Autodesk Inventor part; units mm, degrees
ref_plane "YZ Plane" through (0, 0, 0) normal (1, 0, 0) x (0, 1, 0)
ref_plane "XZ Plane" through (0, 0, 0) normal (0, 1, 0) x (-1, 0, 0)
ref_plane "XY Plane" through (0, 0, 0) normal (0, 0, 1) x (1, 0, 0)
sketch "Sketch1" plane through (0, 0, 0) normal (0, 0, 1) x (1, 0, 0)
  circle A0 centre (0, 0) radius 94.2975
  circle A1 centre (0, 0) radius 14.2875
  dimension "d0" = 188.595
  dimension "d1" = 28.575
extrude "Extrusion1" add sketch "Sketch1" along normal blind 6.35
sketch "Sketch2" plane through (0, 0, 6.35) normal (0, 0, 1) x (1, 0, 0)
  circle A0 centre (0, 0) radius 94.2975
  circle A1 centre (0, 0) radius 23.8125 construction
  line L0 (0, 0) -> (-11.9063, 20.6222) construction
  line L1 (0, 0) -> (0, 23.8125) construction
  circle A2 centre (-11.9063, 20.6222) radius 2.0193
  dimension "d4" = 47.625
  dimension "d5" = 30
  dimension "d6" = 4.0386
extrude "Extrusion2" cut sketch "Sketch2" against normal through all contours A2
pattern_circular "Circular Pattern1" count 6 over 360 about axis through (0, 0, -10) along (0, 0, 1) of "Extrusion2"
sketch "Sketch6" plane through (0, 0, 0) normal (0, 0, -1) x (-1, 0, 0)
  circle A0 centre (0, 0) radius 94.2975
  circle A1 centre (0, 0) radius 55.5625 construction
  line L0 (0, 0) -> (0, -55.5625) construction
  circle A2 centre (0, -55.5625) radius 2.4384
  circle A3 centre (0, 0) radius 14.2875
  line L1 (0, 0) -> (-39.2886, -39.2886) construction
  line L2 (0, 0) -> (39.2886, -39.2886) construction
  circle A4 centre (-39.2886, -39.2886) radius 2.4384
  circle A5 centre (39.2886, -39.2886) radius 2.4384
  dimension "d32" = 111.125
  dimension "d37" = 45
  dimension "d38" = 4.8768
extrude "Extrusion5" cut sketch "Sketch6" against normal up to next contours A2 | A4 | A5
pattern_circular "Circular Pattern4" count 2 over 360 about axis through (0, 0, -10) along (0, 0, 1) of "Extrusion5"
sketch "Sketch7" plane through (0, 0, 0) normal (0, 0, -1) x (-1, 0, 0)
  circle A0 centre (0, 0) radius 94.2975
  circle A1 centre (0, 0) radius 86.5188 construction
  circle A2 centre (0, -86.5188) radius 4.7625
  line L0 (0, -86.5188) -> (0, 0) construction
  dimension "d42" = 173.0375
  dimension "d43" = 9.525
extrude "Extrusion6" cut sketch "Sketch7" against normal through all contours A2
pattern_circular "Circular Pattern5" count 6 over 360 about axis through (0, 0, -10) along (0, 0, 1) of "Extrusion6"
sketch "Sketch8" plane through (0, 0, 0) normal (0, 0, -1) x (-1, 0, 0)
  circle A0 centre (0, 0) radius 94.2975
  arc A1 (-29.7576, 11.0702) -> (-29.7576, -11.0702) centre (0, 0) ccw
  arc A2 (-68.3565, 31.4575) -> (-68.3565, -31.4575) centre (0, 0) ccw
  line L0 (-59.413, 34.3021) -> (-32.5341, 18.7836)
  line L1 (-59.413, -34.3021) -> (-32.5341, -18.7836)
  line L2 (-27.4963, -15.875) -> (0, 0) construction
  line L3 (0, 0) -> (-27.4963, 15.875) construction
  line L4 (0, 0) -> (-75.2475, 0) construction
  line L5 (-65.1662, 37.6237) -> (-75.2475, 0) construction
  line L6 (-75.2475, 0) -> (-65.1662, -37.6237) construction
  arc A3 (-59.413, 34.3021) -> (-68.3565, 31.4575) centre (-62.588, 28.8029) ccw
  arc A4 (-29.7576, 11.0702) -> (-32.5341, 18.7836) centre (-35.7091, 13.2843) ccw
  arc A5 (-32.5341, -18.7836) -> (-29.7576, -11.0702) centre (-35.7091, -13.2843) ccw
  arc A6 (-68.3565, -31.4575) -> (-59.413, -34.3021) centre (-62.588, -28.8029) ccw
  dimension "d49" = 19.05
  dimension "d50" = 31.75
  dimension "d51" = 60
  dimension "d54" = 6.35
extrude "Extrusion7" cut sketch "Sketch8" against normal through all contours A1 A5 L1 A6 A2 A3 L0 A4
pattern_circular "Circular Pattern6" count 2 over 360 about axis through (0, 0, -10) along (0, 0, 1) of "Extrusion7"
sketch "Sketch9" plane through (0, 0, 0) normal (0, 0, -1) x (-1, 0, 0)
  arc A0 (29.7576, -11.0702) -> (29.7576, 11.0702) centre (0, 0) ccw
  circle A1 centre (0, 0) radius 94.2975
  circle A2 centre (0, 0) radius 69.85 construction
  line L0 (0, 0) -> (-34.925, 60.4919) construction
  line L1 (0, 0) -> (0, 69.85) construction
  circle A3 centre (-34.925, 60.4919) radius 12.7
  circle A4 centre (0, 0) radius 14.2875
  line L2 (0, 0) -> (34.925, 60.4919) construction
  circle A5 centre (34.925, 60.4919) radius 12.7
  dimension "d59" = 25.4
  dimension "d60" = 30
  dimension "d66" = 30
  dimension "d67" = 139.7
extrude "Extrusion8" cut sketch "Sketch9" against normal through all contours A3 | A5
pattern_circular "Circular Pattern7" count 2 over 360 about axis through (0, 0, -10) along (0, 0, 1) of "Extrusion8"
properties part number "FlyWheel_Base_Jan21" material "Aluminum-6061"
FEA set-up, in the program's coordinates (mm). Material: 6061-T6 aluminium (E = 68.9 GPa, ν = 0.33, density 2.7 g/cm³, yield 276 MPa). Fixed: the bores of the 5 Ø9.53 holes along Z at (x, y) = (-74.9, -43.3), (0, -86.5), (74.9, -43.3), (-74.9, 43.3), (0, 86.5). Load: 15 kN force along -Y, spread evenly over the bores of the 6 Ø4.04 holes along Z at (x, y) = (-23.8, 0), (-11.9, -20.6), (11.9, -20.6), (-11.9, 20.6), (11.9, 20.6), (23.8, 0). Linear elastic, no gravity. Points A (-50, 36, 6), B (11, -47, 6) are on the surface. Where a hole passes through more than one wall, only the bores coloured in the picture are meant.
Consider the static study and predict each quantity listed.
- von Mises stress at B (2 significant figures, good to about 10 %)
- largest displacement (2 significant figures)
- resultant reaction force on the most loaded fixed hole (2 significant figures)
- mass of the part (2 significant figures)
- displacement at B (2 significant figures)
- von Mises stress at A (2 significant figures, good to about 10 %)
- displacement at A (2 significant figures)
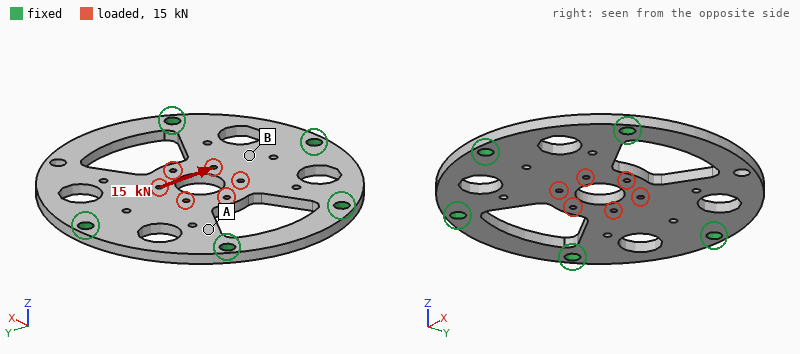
23 MPa
27 µm
5.8 kN
340 g
16 µm
7.1 MPa
8.6 µm
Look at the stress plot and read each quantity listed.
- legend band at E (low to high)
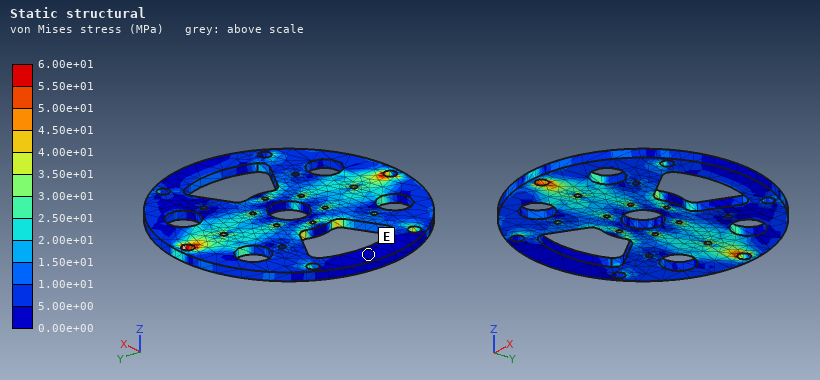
0.00e+00 to 5.00e+00 MPa
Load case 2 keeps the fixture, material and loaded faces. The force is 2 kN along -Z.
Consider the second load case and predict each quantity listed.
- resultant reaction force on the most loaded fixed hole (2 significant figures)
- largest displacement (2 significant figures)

530 N
0.38 mm
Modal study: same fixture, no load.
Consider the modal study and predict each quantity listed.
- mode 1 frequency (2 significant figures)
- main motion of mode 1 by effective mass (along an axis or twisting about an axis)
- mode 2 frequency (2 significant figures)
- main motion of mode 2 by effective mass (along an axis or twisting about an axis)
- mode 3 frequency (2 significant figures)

1100 Hz
along Z
1600 Hz
along Z
2900 Hz
